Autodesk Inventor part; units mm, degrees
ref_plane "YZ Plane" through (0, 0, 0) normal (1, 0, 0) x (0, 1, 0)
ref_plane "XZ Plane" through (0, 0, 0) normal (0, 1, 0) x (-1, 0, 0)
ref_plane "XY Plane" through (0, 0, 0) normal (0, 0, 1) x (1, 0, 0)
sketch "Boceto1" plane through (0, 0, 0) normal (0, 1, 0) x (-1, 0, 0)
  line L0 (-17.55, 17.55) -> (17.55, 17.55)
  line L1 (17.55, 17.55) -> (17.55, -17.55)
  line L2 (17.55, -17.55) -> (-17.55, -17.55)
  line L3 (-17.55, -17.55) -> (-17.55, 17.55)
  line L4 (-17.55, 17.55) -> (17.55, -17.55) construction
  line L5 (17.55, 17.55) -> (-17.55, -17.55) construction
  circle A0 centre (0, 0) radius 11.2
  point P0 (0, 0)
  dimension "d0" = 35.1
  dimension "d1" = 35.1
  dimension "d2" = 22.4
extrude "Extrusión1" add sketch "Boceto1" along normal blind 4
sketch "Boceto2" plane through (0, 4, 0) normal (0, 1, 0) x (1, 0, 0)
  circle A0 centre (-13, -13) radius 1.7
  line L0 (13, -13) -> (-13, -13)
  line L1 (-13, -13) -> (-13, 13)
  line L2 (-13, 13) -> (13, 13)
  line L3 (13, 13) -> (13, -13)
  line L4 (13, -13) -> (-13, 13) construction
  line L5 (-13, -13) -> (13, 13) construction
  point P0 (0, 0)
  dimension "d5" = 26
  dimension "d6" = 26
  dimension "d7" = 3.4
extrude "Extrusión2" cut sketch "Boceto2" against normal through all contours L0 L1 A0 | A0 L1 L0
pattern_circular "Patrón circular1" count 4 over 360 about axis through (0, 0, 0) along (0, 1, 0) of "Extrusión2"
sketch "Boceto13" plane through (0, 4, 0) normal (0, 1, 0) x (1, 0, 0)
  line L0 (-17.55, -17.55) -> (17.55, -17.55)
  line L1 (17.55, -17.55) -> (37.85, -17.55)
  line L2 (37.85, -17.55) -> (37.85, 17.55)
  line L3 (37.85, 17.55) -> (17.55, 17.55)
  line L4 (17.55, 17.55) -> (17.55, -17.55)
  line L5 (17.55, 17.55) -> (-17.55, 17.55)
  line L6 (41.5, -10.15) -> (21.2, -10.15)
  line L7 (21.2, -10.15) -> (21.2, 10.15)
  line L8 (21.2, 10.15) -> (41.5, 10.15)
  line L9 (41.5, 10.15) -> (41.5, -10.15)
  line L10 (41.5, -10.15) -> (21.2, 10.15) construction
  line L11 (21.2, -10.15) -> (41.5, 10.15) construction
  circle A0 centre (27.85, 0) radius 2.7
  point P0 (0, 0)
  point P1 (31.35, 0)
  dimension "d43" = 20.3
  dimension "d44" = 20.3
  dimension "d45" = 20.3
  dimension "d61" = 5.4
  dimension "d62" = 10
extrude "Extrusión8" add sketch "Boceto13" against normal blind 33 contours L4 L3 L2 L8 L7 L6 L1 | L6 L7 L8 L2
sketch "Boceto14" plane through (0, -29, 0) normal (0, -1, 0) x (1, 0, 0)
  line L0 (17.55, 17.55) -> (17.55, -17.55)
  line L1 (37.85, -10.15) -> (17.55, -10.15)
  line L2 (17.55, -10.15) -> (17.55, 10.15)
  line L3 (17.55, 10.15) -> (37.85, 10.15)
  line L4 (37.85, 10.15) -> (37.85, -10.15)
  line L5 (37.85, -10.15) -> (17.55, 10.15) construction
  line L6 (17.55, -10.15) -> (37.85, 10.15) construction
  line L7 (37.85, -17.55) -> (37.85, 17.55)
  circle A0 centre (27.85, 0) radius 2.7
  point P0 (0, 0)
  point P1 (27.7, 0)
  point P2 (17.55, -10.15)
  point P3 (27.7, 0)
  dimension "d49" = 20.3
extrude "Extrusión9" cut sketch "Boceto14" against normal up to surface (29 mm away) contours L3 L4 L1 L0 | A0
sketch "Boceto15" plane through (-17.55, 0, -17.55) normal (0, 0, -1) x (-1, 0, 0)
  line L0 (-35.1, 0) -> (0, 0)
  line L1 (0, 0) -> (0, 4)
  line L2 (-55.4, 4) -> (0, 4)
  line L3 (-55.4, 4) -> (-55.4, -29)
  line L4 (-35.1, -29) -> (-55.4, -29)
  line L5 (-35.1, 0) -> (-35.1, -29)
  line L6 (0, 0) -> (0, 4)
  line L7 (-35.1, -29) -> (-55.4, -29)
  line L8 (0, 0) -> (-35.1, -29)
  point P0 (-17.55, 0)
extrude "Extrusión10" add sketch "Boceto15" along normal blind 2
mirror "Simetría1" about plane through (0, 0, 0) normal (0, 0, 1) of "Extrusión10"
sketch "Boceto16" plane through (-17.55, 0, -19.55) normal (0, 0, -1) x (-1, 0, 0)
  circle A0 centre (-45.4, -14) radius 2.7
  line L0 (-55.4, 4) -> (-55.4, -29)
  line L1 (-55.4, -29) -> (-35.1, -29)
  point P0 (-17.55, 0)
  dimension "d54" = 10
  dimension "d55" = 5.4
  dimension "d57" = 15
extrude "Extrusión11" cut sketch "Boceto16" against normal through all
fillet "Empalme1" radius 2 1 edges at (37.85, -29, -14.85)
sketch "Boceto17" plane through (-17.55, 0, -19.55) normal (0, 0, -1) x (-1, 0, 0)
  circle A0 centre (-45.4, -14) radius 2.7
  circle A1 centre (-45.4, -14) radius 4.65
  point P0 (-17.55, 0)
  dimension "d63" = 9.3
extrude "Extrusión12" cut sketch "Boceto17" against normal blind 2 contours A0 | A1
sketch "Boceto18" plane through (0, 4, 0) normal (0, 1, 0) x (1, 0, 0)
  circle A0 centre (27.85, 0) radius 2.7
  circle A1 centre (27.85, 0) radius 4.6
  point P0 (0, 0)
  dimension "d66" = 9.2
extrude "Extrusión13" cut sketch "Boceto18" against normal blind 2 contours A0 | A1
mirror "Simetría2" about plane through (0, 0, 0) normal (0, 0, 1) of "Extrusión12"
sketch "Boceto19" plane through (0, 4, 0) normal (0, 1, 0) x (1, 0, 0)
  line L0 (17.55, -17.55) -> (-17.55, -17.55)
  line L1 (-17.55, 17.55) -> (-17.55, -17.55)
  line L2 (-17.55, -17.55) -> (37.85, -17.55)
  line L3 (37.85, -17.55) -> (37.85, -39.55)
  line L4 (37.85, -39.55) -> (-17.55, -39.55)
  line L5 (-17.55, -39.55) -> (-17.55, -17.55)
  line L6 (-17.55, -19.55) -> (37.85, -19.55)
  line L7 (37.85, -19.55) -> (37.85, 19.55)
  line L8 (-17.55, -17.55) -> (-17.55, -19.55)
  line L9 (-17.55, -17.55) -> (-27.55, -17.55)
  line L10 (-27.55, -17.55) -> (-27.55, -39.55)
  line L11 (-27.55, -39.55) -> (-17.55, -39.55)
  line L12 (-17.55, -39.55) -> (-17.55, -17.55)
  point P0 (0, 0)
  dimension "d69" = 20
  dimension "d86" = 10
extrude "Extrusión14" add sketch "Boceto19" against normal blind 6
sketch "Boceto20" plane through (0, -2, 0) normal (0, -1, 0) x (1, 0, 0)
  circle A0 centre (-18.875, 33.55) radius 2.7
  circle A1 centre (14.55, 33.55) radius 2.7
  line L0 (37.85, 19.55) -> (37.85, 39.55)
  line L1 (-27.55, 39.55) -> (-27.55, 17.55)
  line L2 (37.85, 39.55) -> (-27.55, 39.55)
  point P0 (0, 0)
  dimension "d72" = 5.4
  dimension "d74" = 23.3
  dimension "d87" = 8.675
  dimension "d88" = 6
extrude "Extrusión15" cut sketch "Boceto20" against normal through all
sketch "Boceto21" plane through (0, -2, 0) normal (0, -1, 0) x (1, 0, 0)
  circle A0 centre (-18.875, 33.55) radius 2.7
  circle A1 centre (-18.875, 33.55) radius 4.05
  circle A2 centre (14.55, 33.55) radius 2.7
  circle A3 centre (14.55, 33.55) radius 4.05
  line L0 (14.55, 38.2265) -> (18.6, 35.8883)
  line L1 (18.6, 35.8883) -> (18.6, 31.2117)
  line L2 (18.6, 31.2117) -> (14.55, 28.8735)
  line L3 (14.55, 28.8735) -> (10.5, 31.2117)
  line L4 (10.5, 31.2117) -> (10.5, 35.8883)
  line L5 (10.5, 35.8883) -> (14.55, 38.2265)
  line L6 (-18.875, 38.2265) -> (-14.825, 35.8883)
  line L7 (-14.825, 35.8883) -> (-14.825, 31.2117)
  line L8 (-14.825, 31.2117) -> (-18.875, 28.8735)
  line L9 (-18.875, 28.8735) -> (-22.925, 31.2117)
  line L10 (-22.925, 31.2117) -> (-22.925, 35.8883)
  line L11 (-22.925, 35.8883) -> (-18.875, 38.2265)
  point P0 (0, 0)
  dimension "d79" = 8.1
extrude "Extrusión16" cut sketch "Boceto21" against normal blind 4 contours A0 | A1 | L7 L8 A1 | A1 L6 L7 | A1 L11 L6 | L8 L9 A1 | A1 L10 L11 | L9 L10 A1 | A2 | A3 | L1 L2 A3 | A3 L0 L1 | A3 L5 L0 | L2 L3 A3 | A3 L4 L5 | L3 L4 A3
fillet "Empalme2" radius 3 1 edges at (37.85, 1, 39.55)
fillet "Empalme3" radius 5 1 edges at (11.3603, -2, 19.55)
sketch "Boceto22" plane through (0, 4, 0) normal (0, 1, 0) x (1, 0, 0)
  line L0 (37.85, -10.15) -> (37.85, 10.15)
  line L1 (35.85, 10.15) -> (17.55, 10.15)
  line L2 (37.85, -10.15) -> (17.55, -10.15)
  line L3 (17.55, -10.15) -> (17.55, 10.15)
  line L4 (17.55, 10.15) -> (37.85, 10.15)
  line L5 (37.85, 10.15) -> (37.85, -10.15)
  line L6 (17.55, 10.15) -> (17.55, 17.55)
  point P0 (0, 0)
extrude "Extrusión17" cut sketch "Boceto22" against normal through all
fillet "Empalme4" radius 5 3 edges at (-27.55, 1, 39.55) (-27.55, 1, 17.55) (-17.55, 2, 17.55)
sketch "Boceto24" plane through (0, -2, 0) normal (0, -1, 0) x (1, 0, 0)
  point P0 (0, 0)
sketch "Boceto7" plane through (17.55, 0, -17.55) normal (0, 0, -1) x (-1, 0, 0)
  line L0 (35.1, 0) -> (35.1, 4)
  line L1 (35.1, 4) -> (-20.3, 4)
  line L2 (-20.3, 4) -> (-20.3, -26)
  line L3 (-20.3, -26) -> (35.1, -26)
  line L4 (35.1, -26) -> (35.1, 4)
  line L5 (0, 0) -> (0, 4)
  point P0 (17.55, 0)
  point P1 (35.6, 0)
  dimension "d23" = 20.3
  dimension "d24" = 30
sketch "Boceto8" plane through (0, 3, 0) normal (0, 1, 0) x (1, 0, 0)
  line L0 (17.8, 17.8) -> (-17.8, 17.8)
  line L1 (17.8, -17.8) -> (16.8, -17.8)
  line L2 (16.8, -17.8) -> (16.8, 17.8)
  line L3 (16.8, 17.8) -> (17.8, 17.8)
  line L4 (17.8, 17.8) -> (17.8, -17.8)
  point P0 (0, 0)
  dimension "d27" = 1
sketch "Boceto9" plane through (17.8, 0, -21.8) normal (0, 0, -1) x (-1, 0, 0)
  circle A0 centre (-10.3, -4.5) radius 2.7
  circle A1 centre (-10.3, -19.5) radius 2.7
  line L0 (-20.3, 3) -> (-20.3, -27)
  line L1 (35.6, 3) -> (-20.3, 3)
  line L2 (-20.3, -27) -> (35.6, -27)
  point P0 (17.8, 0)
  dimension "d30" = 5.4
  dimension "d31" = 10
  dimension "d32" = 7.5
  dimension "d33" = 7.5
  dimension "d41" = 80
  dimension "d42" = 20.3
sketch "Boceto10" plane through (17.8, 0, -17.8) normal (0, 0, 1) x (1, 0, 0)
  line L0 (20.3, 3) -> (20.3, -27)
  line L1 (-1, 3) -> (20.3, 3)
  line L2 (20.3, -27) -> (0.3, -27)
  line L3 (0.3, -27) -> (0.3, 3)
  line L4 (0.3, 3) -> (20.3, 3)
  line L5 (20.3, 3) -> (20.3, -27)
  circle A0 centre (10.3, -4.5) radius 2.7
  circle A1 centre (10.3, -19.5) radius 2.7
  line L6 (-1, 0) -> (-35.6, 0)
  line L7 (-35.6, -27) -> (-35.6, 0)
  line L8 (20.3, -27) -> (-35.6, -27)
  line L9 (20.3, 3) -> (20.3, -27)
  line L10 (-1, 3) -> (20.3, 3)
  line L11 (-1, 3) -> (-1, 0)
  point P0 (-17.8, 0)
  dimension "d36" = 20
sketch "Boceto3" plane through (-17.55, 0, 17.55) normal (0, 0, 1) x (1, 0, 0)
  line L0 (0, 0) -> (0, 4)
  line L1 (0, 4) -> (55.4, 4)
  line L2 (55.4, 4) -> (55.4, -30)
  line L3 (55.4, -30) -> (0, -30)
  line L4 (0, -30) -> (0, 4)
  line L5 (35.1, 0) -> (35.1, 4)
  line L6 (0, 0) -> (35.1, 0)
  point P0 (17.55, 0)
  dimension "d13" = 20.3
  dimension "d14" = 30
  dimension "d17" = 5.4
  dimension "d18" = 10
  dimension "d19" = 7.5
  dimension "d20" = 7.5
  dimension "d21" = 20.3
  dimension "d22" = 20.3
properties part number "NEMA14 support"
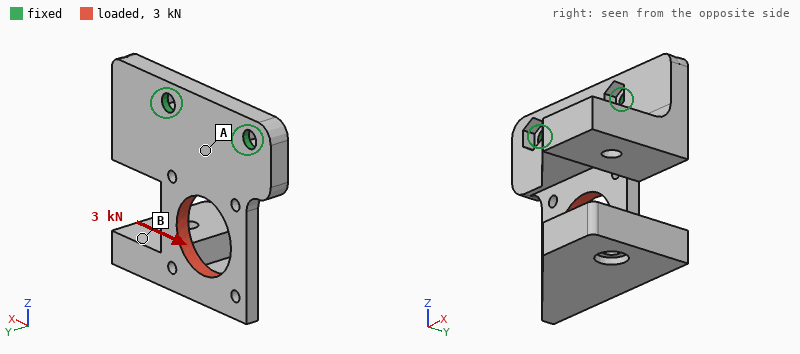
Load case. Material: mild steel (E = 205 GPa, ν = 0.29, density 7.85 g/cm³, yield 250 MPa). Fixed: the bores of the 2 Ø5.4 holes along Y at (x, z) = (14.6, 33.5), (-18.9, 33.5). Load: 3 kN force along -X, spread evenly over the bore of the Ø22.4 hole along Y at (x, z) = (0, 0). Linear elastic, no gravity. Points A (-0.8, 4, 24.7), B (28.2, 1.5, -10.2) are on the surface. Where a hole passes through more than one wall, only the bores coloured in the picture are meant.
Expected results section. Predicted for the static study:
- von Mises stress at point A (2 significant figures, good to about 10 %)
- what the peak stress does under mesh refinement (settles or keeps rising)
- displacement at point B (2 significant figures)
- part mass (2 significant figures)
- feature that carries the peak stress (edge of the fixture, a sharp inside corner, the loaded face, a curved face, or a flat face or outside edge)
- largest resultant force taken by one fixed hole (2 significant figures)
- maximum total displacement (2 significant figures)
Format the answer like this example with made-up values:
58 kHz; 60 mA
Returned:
44 MPa; keeps rising; 50 µm; 200 g; edge of the fixture; 3.2 kN; 60 µm
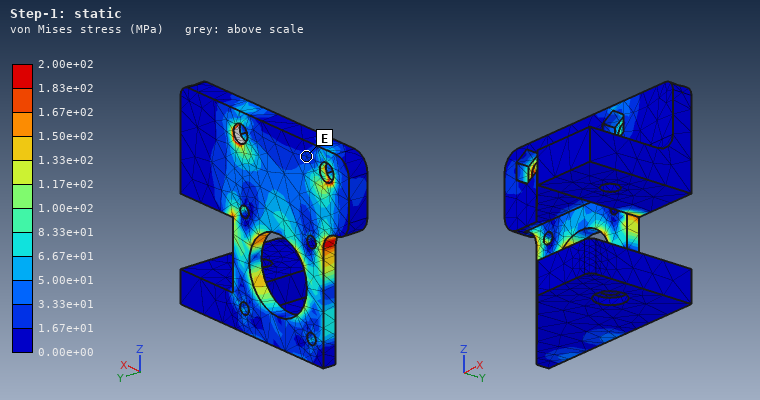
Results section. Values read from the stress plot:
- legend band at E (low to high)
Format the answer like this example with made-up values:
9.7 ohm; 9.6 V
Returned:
1.67e+01 to 3.33e+01 MPa
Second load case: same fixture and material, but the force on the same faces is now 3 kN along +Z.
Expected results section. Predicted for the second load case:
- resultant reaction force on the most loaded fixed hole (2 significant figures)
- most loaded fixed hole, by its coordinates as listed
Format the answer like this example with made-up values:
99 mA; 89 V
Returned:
1.7 kN; (14.6, 33.5)
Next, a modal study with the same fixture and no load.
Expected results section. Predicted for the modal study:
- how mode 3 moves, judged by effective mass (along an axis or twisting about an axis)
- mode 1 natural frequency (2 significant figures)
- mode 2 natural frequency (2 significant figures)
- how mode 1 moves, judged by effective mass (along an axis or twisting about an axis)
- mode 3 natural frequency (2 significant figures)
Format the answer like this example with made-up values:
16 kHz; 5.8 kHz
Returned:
along Y; 480 Hz; 1000 Hz; along Y; 1500 Hz
